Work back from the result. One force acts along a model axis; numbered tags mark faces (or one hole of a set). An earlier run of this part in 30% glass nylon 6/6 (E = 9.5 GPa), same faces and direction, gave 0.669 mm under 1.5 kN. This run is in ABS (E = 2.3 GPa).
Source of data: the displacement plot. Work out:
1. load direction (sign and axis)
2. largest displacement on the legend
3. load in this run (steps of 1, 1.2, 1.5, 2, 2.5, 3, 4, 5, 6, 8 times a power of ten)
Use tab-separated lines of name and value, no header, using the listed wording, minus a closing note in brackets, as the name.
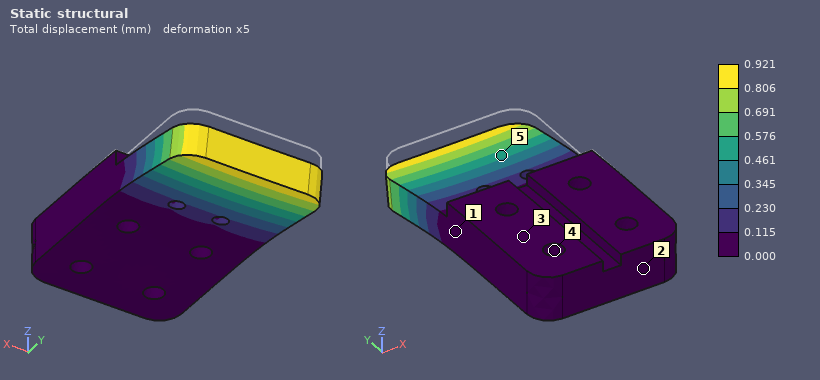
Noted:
load direction	-Z
largest displacement on the legend	0.921 mm
load in this run	500 N
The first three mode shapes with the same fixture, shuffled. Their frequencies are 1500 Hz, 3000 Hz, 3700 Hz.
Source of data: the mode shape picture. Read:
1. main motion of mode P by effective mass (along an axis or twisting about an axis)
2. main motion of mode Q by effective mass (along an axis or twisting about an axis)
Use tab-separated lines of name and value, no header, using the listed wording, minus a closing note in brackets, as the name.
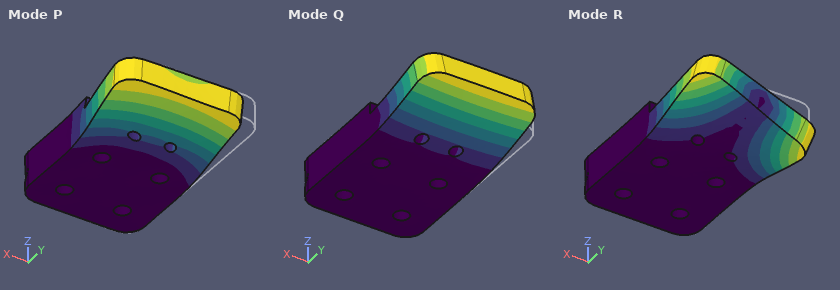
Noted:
main motion of mode P by effective mass	along X
main motion of mode Q by effective mass	along Z
